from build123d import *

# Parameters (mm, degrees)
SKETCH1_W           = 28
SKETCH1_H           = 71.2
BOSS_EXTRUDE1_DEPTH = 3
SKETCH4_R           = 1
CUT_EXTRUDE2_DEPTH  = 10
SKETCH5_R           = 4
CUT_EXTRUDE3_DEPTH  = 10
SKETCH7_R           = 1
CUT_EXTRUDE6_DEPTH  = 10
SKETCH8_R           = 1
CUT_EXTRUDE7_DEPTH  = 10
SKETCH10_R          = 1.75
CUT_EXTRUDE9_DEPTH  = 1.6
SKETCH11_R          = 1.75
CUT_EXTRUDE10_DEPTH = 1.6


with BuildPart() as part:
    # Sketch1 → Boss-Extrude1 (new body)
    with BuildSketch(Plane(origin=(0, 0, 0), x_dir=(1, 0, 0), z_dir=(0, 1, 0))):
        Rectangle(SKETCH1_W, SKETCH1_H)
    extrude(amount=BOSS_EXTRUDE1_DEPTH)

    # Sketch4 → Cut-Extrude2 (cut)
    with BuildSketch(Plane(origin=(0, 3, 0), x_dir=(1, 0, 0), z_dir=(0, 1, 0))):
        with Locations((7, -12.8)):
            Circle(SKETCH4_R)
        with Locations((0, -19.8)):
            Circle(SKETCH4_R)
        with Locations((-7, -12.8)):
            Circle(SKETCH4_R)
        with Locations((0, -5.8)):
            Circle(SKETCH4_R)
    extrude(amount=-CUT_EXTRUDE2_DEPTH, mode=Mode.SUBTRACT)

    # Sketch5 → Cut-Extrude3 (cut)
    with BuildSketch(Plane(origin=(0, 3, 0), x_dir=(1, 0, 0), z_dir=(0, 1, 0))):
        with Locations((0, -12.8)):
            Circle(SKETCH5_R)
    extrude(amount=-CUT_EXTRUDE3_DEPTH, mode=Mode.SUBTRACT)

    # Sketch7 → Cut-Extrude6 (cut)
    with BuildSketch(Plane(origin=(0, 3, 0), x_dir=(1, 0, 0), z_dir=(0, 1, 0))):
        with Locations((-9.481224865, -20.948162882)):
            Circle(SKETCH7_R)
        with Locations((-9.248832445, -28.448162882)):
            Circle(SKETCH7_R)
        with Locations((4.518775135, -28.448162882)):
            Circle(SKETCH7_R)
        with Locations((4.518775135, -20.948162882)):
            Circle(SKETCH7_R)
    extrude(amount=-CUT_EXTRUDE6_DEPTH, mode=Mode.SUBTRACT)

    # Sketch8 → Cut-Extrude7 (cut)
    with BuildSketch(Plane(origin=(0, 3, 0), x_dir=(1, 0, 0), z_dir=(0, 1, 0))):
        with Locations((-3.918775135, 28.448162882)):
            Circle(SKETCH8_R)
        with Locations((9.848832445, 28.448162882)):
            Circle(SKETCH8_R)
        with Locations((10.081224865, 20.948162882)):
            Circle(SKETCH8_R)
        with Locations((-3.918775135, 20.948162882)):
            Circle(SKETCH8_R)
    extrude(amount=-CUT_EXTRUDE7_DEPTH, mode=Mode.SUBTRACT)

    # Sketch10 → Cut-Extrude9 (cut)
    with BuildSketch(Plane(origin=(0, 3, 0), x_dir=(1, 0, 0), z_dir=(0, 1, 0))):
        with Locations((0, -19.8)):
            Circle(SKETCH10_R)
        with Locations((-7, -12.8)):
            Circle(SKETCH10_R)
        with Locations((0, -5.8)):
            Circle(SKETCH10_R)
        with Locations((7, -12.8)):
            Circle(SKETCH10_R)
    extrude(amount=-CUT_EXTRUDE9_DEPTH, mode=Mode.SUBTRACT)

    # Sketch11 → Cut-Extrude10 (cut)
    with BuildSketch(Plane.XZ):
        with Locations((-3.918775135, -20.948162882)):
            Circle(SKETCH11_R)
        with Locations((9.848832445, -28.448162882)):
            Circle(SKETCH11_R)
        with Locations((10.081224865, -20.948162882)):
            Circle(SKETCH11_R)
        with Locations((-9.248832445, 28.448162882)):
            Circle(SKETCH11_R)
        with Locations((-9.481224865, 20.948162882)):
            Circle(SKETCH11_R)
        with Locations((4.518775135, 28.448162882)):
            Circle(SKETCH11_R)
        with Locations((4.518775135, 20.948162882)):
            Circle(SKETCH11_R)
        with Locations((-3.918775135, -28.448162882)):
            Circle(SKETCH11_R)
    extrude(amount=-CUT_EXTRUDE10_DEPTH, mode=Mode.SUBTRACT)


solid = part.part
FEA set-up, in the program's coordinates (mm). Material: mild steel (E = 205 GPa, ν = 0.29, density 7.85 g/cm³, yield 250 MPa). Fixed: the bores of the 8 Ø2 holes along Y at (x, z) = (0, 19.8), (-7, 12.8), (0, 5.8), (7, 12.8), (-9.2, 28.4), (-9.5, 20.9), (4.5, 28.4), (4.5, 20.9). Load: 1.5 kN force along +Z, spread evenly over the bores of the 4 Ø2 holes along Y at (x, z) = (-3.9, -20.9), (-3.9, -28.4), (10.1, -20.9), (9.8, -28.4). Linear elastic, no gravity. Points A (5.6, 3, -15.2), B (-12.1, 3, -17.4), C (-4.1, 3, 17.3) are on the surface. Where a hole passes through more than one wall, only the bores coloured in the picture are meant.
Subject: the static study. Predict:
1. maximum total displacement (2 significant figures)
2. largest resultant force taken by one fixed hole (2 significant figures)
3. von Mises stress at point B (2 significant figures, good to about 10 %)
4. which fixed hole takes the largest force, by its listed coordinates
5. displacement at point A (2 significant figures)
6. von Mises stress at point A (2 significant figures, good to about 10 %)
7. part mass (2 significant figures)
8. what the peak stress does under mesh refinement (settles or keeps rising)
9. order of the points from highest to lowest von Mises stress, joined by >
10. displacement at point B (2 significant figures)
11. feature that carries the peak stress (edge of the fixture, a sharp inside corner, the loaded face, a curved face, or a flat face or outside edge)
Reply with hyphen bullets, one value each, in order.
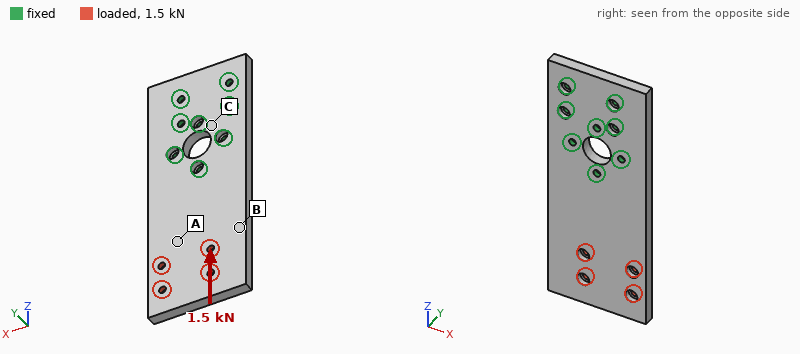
- 98 µm
- 550 N
- 30 MPa
- (7, 12.8)
- 34 µm
- 49 MPa
- 44 g
- keeps rising
- A > B > C
- 36 µm
- edge of the fixture
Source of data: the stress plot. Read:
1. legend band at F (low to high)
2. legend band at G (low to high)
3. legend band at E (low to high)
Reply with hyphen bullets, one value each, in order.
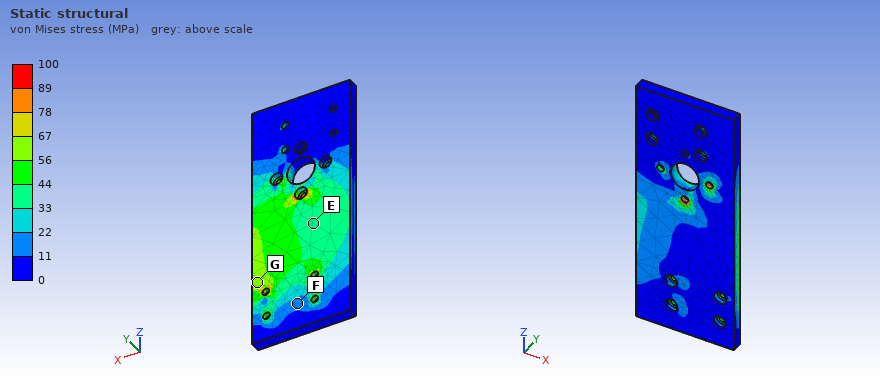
- 11 to 22 MPa
- 56 to 67 MPa
- 33 to 44 MPa
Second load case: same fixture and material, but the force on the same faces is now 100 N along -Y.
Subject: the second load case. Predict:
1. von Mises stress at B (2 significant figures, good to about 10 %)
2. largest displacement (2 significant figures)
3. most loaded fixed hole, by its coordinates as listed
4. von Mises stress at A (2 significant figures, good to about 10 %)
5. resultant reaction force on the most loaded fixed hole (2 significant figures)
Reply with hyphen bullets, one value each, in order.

- 20 MPa
- 0.16 mm
- (0, 5.8)
- 21 MPa
- 490 N
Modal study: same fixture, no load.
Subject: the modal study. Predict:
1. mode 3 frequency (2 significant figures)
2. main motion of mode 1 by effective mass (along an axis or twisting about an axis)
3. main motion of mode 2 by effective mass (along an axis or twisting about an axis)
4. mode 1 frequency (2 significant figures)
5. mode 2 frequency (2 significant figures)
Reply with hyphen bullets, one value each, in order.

- 7100 Hz
- along Y
- twisting about Z
- 1300 Hz
- 3700 Hz
